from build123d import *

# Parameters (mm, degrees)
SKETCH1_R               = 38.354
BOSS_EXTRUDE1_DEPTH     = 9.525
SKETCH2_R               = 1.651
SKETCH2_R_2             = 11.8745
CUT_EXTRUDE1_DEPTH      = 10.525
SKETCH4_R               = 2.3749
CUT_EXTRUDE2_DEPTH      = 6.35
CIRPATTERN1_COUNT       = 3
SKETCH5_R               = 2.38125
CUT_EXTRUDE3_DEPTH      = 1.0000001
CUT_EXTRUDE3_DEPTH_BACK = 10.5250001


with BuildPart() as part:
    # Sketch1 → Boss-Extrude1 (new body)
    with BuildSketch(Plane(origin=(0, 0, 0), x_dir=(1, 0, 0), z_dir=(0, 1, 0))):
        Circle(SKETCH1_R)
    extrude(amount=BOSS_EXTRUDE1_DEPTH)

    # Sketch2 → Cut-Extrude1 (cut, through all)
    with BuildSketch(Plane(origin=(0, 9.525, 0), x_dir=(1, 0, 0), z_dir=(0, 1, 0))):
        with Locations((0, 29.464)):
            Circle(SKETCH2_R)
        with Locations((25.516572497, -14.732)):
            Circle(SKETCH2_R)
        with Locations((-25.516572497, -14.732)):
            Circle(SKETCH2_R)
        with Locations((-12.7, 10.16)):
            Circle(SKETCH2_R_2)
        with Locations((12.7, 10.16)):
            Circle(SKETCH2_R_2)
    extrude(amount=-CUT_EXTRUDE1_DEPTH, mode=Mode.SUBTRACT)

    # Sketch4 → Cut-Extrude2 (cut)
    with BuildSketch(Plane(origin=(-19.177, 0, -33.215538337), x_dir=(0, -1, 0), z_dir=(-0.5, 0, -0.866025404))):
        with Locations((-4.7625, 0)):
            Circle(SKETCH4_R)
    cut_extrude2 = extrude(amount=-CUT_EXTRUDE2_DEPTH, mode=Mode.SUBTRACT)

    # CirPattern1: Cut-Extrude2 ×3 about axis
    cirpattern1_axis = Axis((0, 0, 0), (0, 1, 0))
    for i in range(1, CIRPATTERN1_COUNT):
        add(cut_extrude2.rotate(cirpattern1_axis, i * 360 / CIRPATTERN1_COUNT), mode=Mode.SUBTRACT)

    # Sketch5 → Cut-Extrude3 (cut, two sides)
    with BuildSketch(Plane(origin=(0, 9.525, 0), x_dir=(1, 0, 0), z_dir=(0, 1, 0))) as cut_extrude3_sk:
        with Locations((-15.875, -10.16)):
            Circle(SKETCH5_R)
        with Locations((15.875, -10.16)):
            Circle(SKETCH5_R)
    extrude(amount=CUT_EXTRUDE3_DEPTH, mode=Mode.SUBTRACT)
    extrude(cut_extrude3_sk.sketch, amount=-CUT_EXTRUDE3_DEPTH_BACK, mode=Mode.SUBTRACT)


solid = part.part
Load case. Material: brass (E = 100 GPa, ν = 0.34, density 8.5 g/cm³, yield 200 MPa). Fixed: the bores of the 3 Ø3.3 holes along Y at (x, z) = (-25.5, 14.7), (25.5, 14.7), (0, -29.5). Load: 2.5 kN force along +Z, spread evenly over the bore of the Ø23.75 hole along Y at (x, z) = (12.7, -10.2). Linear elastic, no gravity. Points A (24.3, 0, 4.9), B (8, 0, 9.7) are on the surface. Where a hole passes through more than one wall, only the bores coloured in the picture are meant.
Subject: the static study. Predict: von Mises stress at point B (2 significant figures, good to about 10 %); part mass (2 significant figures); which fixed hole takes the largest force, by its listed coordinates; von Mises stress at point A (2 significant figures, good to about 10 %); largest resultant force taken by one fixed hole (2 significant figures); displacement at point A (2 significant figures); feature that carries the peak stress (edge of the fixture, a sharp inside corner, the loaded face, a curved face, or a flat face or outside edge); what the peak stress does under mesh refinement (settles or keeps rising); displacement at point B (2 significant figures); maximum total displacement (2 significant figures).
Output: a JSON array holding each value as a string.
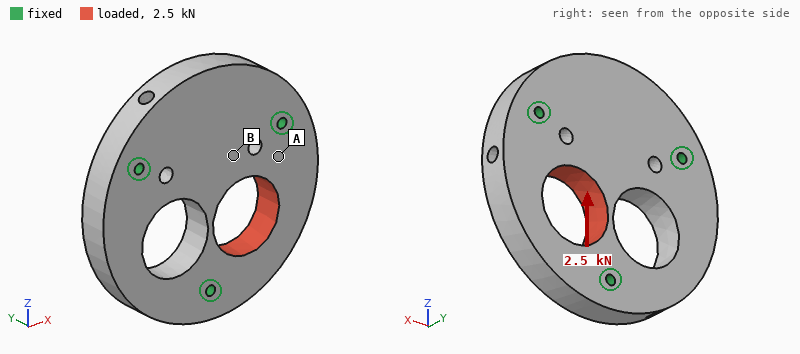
["2.9 MPa", "290 g", "(25.5, 14.7)", "8.6 MPa", "1.4 kN", "0.96 µm", "edge of the fixture", "keeps rising", "1.3 µm", "3.2 µm"]
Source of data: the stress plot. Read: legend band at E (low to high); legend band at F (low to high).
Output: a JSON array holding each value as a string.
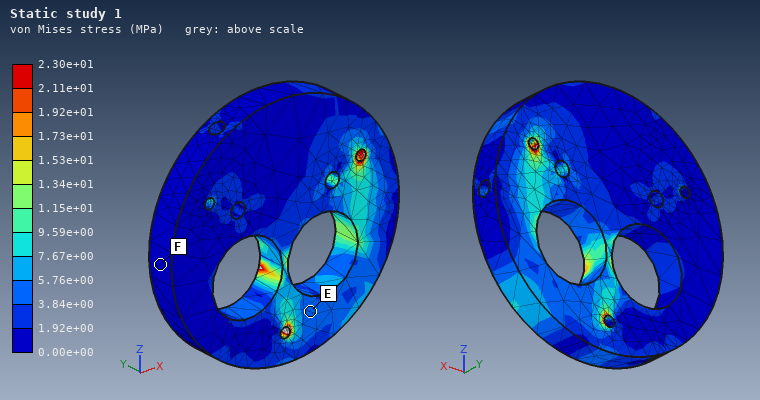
["3.84e+00 to 5.76e+00 MPa", "0.00e+00 to 1.92e+00 MPa"]
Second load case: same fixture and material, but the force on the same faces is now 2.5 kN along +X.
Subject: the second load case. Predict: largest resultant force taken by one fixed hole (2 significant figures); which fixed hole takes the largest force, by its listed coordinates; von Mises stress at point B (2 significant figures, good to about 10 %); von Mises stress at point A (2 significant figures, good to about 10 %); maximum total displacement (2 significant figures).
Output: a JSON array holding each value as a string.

["1.3 kN", "(0, -29.5)", "5.3 MPa", "4.1 MPa", "5.0 µm"]
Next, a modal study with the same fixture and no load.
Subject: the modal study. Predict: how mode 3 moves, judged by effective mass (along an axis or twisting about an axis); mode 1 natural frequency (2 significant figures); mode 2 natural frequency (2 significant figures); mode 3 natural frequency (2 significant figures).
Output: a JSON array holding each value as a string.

["along Y", "5800 Hz", "5900 Hz", "7000 Hz"]
